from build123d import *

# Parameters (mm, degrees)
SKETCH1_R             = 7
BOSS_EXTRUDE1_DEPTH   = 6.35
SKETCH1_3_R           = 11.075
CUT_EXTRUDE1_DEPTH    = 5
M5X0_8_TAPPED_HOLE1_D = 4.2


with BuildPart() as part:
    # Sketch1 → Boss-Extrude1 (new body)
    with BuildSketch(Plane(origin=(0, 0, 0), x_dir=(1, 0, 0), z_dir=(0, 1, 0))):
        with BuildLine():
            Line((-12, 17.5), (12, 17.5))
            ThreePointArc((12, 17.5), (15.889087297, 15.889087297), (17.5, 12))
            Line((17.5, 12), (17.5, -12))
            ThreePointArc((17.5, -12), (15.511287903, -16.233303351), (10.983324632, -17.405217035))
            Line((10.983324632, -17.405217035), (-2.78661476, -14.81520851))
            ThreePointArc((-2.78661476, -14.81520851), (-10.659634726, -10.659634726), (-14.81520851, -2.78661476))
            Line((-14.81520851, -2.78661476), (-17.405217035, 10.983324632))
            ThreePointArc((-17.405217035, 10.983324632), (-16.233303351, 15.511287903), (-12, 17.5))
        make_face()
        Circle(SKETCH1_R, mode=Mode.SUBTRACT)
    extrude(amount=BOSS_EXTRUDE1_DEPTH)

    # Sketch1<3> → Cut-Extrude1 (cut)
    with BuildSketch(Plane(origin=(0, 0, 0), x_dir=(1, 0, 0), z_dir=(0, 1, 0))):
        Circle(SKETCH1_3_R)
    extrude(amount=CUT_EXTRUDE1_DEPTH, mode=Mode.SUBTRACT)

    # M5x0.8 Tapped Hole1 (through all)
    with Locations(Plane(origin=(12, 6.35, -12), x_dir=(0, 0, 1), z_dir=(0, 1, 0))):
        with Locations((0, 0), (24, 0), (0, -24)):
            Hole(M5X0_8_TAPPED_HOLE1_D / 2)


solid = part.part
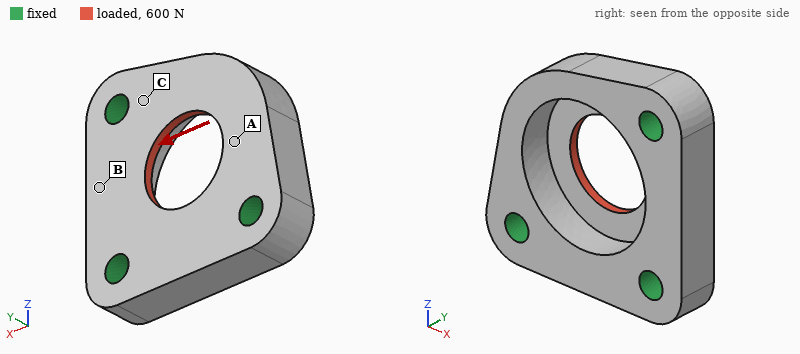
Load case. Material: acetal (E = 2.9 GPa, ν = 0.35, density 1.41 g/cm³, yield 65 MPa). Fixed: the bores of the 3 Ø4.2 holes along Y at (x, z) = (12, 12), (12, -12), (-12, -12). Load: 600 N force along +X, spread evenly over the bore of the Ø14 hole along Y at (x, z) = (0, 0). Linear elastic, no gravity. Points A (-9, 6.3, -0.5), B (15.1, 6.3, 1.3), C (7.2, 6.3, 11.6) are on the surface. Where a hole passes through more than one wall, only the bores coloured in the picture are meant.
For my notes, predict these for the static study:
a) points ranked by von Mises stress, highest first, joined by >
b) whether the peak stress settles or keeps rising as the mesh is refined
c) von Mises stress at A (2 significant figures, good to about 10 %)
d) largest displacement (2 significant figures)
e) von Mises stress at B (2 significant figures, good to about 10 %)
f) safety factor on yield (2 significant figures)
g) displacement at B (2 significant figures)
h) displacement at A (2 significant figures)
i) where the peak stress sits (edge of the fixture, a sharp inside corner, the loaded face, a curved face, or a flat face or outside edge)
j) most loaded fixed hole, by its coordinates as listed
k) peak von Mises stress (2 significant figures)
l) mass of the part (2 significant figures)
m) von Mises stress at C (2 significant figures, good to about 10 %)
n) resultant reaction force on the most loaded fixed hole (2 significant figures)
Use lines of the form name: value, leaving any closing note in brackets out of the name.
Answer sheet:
points ranked by von Mises stress, highest first, joined by >: A > C > B
whether the peak stress settles or keeps rising as the mesh is refined: settles
von Mises stress at A: 12 MPa
largest displacement: 91 µm
von Mises stress at B: 2.7 MPa
safety factor on yield: 3.0
displacement at B: 28 µm
displacement at A: 69 µm
where the peak stress sits: the loaded face
most loaded fixed hole, by its coordinates as listed: (12, 12)
peak von Mises stress: 22 MPa
mass of the part: 6.1 g
von Mises stress at C: 8.5 MPa
resultant reaction force on the most loaded fixed hole: 270 N
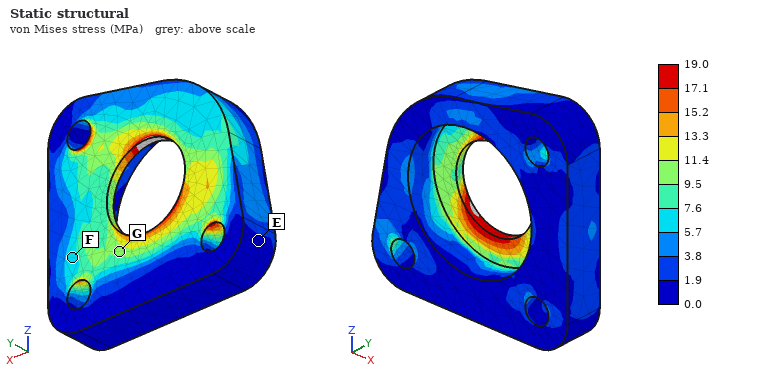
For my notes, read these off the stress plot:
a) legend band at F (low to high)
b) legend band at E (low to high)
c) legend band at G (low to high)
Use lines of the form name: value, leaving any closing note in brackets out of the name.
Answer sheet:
legend band at F: 5.7 to 7.6 MPa
legend band at E: 0.0 to 1.9 MPa
legend band at G: 9.5 to 11.4 MPa
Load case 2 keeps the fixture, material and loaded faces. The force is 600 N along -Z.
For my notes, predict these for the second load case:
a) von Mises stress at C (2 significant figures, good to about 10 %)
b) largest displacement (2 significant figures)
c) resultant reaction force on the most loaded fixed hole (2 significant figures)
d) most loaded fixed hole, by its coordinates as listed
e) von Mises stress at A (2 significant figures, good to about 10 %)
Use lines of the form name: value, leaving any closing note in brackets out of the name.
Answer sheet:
von Mises stress at C: 9.9 MPa
largest displacement: 91 µm
resultant reaction force on the most loaded fixed hole: 270 N
most loaded fixed hole, by its coordinates as listed: (-12, -12)
von Mises stress at A: 11 MPa
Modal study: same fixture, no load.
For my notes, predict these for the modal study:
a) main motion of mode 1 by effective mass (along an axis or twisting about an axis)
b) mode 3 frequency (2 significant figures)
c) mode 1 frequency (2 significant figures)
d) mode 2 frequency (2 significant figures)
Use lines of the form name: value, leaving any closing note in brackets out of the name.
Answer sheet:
main motion of mode 1 by effective mass: along Y
mode 3 frequency: 12 kHz
mode 1 frequency: 4800 Hz
mode 2 frequency: 10 kHz
